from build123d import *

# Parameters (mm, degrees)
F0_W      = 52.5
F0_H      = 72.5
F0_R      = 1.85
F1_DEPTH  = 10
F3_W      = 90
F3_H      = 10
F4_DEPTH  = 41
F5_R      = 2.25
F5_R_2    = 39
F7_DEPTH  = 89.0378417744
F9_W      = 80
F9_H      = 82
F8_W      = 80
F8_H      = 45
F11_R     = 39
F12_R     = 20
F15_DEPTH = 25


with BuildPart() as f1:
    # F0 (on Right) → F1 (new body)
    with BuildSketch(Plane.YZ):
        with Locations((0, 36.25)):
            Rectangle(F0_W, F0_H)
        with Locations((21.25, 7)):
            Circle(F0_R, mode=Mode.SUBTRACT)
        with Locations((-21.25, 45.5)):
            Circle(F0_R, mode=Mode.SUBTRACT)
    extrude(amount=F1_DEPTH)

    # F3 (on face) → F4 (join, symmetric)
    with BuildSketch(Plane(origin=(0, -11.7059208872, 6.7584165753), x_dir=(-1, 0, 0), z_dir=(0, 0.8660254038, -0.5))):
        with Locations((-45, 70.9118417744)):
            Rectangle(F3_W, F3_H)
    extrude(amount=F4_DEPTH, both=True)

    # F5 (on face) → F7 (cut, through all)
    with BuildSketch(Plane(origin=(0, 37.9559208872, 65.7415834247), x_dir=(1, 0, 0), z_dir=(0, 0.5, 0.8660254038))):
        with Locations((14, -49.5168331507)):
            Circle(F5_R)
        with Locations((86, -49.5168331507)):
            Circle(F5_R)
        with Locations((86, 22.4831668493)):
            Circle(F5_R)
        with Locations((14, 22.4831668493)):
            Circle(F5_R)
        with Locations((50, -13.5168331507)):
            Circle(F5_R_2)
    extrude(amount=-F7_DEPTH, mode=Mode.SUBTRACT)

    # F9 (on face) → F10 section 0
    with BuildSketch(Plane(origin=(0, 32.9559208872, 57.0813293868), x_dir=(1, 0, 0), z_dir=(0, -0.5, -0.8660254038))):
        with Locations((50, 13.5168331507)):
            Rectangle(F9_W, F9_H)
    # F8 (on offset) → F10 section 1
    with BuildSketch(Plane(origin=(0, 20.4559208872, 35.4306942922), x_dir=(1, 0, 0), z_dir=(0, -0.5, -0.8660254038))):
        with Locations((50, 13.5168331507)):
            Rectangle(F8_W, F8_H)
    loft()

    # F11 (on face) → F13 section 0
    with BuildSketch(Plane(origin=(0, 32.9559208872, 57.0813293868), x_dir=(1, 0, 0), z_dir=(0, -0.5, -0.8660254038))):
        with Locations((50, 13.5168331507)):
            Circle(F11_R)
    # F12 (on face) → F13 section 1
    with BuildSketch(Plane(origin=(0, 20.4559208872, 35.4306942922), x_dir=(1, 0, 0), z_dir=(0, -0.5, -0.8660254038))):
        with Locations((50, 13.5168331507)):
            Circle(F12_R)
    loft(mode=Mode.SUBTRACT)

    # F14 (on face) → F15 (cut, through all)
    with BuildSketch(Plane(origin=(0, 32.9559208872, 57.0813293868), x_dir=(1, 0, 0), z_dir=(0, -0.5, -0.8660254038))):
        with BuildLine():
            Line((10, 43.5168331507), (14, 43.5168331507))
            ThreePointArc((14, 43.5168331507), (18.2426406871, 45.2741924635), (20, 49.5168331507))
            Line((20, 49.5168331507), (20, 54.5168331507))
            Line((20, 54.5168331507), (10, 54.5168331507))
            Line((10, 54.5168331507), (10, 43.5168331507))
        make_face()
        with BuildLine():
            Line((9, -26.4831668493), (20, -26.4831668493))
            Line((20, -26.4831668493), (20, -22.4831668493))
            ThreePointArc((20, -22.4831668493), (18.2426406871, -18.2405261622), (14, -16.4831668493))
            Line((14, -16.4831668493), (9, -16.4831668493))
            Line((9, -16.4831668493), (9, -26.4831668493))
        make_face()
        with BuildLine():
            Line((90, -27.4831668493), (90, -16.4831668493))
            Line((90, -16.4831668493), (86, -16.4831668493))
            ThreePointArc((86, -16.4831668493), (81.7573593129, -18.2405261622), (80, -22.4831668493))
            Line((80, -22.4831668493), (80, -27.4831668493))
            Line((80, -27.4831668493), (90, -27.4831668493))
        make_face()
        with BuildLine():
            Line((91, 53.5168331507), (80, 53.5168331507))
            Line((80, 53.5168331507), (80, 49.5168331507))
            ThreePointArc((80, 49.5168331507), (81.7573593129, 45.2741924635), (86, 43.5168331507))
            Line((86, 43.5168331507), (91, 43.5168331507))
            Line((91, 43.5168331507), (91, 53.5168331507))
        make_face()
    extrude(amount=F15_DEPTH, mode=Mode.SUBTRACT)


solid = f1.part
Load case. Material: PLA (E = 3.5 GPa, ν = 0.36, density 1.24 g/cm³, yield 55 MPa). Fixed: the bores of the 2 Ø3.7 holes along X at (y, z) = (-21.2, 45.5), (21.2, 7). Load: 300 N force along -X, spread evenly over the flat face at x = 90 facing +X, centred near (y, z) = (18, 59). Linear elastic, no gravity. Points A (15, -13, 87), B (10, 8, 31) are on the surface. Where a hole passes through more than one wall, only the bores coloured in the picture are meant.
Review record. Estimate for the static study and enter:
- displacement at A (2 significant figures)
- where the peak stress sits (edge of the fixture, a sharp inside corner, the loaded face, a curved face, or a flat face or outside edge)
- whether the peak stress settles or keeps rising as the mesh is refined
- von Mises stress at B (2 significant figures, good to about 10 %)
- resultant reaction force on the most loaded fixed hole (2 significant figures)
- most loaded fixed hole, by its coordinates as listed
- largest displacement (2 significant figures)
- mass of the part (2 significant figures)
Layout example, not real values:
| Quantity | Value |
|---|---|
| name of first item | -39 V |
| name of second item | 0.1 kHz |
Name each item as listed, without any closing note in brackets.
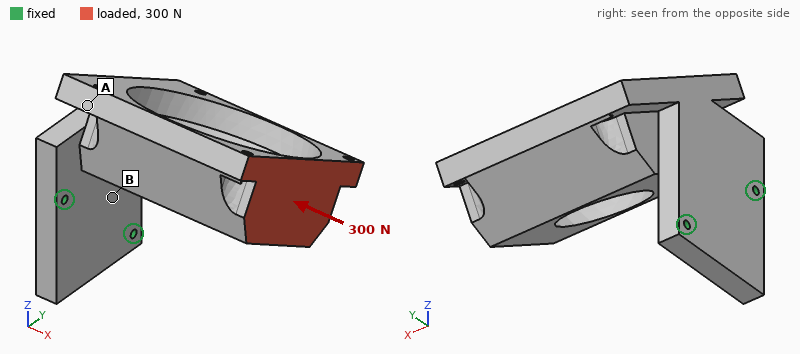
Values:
| Quantity | Value |
|---|---|
| displacement at A | 0.47 mm |
| where the peak stress sits | edge of the fixture |
| whether the peak stress settles or keeps rising as the mesh is refined | keeps rising |
| von Mises stress at B | 5.2 MPa |
| resultant reaction force on the most loaded fixed hole | 180 N |
| most loaded fixed hole, by its coordinates as listed | (-21.2, 45.5) |
| largest displacement | 1.7 mm |
| mass of the part | 140 g |
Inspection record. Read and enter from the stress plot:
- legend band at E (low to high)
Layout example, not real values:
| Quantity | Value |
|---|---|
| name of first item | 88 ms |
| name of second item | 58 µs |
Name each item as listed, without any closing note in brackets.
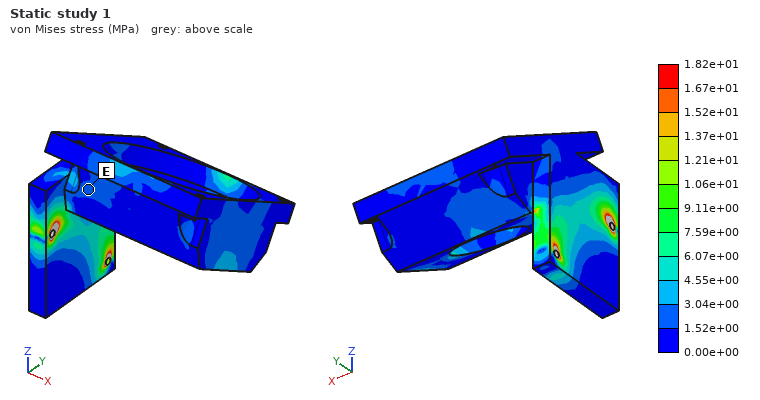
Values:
| Quantity | Value |
|---|---|
| legend band at E | 1.52e+00 to 3.04e+00 MPa |
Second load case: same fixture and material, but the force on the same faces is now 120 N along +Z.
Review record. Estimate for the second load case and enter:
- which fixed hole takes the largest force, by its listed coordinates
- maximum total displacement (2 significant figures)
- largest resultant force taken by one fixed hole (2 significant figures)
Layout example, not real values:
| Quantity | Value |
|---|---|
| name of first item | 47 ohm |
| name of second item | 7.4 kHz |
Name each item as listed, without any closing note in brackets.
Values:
| Quantity | Value |
|---|---|
| which fixed hole takes the largest force, by its listed coordinates | (21.2, 7) |
| maximum total displacement | 1.7 mm |
| largest resultant force taken by one fixed hole | 150 N |
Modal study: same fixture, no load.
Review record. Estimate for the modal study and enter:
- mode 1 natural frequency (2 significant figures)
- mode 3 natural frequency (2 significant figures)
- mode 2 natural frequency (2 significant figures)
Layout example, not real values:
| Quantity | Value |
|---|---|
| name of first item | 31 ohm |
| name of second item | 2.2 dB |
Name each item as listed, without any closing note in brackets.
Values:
| Quantity | Value |
|---|---|
| mode 1 natural frequency | 190 Hz |
| mode 3 natural frequency | 700 Hz |
| mode 2 natural frequency | 340 Hz |
